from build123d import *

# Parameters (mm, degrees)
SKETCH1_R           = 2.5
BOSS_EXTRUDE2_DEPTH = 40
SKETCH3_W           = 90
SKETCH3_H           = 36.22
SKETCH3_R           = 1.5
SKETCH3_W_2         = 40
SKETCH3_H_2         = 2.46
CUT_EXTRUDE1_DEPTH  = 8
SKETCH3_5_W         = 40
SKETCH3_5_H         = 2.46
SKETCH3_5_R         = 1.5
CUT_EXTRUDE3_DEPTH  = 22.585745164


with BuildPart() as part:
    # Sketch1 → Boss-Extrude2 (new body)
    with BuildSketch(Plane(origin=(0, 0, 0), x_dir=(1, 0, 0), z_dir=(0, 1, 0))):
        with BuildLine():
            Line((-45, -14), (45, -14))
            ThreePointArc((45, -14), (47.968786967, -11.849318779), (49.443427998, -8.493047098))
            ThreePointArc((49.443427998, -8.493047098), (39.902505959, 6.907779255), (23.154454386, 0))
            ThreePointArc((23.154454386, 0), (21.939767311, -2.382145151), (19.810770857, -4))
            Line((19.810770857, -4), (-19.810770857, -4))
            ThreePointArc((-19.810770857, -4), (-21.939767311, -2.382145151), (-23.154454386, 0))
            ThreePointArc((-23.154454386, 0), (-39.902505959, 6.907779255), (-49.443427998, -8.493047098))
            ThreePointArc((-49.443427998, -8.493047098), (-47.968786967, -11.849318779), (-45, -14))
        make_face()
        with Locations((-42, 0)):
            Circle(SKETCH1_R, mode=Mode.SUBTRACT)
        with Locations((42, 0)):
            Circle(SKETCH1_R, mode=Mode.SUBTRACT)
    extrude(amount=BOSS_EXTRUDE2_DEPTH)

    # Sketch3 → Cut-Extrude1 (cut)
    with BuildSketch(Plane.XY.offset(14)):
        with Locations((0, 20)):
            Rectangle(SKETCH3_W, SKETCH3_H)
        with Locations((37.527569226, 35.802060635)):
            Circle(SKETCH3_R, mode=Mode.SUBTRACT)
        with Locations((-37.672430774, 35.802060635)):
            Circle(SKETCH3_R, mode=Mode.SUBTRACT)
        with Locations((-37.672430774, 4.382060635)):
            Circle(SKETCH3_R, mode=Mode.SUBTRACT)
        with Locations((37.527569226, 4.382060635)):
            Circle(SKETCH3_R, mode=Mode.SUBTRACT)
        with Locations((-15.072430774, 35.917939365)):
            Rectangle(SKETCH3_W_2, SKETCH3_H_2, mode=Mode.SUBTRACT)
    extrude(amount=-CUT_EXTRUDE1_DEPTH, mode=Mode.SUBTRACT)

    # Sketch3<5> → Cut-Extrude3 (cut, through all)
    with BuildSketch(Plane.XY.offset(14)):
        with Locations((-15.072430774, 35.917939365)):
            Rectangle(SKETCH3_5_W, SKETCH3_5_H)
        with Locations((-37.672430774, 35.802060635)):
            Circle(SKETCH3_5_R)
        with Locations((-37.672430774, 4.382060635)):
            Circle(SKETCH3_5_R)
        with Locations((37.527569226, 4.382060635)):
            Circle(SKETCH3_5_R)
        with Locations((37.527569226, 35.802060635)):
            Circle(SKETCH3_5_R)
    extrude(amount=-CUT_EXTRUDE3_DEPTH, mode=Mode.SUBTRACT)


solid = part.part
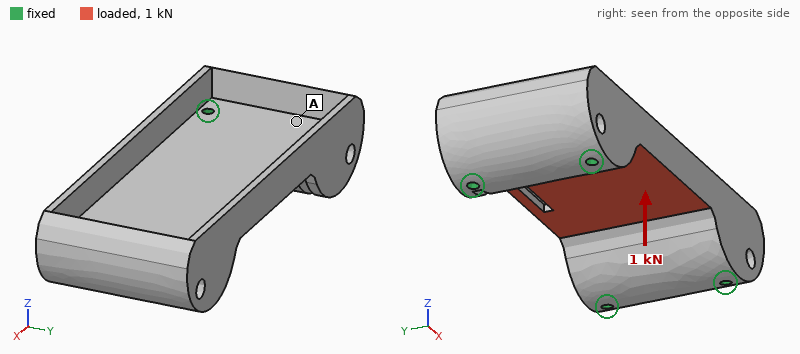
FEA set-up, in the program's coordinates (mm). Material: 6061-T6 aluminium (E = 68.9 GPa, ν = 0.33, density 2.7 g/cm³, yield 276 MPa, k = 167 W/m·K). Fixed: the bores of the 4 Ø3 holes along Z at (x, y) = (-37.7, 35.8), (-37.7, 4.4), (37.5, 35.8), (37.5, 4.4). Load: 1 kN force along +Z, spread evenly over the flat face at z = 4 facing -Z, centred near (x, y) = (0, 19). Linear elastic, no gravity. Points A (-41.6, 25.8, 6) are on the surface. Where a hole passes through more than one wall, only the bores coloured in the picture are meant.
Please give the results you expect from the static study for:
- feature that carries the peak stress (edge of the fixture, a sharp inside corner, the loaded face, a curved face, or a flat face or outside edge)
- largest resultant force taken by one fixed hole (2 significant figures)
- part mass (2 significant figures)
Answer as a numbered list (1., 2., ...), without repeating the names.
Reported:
1. a flat face or outside edge
2. 390 N
3. 81 g
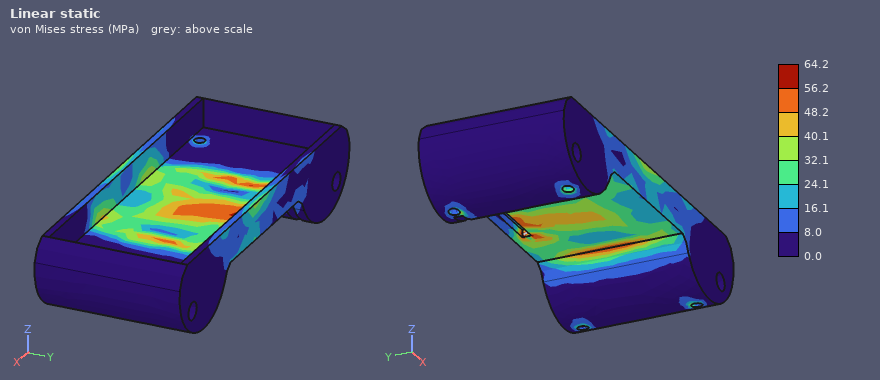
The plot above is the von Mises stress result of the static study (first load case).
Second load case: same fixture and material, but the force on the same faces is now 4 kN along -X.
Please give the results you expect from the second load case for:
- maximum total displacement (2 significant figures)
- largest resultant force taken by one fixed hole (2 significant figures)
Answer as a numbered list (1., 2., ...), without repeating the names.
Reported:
1. 15 µm
2. 1.1 kN
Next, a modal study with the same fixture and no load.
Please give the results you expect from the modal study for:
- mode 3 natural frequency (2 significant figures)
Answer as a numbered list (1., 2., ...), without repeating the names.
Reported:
1. 12 kHz
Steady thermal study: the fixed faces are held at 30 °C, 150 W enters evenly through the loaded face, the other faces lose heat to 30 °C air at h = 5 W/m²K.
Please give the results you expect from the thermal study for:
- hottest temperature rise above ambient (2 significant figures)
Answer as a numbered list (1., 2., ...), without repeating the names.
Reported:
1. 84 K
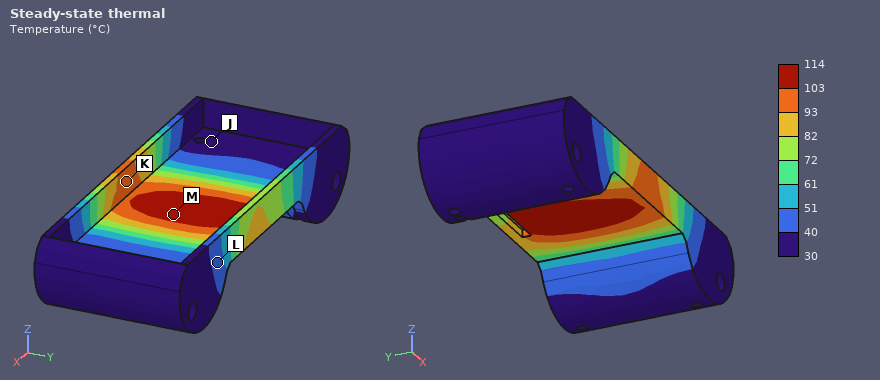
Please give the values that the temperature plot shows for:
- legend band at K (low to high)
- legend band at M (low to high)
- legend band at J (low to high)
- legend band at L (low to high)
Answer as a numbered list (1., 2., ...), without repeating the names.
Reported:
1. 93 to 103 °C
2. 103 to 114 °C
3. 30 to 40 °C
4. 40 to 51 °C
